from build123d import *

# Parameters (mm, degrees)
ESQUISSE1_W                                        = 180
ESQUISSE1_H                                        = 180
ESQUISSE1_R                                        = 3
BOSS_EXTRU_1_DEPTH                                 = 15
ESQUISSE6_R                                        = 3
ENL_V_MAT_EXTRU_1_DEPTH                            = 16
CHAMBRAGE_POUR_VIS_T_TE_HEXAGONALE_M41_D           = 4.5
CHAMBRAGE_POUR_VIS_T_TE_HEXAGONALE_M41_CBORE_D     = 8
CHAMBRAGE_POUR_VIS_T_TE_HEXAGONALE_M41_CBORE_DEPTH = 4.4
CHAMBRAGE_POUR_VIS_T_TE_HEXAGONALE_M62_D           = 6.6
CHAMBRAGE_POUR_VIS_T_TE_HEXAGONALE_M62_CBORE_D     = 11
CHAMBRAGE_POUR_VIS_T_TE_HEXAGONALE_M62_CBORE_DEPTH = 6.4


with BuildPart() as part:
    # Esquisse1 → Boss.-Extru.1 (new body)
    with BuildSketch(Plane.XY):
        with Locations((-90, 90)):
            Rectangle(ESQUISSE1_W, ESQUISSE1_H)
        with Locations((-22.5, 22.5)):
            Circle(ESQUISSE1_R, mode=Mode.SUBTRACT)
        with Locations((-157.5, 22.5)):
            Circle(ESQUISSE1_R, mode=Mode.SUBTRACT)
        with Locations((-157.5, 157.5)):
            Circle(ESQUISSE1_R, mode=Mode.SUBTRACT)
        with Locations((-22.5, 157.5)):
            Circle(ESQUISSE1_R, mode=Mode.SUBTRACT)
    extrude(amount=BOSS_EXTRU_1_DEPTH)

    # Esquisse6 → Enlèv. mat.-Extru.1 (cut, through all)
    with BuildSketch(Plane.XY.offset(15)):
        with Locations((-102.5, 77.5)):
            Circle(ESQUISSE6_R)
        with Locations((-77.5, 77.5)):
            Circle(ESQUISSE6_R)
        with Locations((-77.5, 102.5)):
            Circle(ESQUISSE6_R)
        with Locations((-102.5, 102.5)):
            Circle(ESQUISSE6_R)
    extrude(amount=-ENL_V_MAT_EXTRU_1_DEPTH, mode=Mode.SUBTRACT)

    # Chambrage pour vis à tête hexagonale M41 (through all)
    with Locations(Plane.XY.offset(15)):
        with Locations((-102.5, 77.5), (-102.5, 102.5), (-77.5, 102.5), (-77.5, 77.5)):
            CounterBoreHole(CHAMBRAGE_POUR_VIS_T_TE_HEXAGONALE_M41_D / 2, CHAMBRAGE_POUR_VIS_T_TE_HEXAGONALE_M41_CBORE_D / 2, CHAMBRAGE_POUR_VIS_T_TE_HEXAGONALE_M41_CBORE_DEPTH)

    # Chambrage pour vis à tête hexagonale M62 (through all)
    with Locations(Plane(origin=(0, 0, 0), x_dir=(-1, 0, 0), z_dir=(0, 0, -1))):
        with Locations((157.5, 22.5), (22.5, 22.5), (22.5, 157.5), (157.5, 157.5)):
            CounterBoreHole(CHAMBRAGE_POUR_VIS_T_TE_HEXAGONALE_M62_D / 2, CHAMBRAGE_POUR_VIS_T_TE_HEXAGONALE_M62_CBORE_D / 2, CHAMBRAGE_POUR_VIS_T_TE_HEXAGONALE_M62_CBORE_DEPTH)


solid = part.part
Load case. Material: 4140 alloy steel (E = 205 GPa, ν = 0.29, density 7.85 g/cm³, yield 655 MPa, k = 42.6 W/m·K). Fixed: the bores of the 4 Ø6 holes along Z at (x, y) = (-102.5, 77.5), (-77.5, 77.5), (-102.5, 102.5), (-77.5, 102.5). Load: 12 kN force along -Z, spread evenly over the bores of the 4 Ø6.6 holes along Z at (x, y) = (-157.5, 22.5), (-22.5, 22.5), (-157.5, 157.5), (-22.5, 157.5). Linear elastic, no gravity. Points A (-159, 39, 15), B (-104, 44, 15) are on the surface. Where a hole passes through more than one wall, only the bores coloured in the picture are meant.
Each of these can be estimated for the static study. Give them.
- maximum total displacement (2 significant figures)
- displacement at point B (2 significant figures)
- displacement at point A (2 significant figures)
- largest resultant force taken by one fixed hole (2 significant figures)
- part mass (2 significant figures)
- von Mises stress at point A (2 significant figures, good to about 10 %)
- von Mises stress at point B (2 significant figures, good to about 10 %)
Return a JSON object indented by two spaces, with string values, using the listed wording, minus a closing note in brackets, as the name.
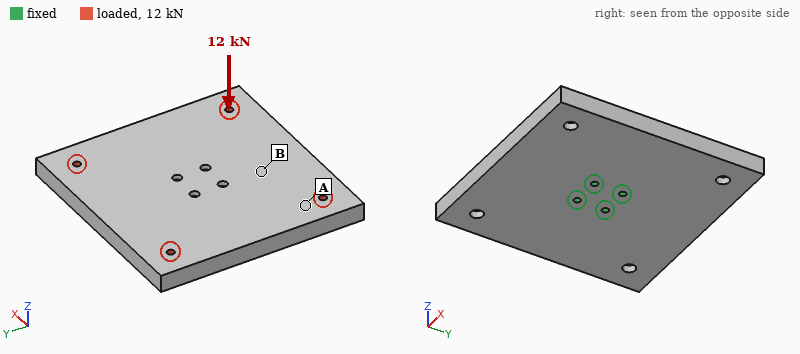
{
  "maximum total displacement": "0.12 mm",
  "displacement at point B": "0.023 mm",
  "displacement at point A": "0.069 mm",
  "largest resultant force taken by one fixed hole": "4.3 kN",
  "part mass": "3.8 kg",
  "von Mises stress at point A": "13 MPa",
  "von Mises stress at point B": "36 MPa"
}
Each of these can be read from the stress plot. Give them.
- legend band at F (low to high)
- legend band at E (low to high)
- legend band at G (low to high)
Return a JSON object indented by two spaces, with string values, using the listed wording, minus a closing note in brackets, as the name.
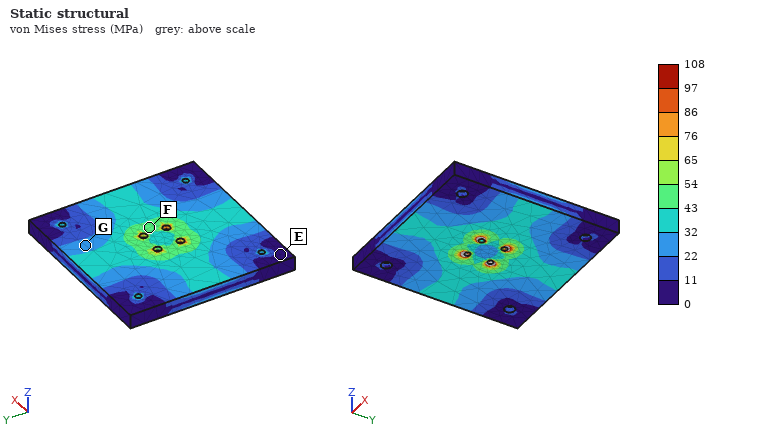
{
  "legend band at F": "43 to 54 MPa",
  "legend band at E": "0 to 11 MPa",
  "legend band at G": "22 to 32 MPa"
}
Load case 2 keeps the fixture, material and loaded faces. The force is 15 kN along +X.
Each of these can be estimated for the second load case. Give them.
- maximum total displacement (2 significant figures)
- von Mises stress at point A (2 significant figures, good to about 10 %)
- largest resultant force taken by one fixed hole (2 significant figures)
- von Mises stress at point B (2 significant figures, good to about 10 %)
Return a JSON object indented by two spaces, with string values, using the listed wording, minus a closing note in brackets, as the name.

{
  "maximum total displacement": "16 µm",
  "von Mises stress at point A": "7.7 MPa",
  "largest resultant force taken by one fixed hole": "3.9 kN",
  "von Mises stress at point B": "7.4 MPa"
}
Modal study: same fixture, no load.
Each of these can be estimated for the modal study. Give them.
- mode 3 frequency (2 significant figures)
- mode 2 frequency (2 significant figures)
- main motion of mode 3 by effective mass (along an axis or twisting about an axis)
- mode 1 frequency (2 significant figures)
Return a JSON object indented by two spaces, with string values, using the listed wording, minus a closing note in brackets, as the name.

{
  "mode 3 frequency": "1500 Hz",
  "mode 2 frequency": "1200 Hz",
  "main motion of mode 3 by effective mass": "along Z",
  "mode 1 frequency": "1200 Hz"
}
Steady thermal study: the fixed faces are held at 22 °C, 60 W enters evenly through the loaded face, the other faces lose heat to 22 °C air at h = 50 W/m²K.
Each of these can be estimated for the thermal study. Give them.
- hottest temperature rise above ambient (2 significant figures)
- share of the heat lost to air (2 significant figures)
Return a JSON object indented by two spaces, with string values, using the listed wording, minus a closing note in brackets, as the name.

{
  "hottest temperature rise above ambient": "25 K",
  "share of the heat lost to air": "63 %"
}
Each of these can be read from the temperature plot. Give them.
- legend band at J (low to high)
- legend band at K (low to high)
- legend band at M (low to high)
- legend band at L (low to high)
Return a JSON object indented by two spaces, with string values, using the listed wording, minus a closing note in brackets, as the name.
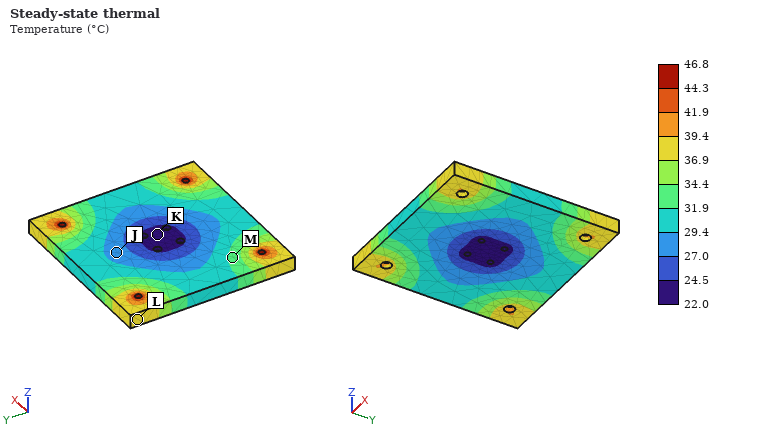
{
  "legend band at J": "27.0 to 29.4 °C",
  "legend band at K": "22.0 to 24.5 °C",
  "legend band at M": "31.9 to 34.4 °C",
  "legend band at L": "36.9 to 39.4 °C"
}
